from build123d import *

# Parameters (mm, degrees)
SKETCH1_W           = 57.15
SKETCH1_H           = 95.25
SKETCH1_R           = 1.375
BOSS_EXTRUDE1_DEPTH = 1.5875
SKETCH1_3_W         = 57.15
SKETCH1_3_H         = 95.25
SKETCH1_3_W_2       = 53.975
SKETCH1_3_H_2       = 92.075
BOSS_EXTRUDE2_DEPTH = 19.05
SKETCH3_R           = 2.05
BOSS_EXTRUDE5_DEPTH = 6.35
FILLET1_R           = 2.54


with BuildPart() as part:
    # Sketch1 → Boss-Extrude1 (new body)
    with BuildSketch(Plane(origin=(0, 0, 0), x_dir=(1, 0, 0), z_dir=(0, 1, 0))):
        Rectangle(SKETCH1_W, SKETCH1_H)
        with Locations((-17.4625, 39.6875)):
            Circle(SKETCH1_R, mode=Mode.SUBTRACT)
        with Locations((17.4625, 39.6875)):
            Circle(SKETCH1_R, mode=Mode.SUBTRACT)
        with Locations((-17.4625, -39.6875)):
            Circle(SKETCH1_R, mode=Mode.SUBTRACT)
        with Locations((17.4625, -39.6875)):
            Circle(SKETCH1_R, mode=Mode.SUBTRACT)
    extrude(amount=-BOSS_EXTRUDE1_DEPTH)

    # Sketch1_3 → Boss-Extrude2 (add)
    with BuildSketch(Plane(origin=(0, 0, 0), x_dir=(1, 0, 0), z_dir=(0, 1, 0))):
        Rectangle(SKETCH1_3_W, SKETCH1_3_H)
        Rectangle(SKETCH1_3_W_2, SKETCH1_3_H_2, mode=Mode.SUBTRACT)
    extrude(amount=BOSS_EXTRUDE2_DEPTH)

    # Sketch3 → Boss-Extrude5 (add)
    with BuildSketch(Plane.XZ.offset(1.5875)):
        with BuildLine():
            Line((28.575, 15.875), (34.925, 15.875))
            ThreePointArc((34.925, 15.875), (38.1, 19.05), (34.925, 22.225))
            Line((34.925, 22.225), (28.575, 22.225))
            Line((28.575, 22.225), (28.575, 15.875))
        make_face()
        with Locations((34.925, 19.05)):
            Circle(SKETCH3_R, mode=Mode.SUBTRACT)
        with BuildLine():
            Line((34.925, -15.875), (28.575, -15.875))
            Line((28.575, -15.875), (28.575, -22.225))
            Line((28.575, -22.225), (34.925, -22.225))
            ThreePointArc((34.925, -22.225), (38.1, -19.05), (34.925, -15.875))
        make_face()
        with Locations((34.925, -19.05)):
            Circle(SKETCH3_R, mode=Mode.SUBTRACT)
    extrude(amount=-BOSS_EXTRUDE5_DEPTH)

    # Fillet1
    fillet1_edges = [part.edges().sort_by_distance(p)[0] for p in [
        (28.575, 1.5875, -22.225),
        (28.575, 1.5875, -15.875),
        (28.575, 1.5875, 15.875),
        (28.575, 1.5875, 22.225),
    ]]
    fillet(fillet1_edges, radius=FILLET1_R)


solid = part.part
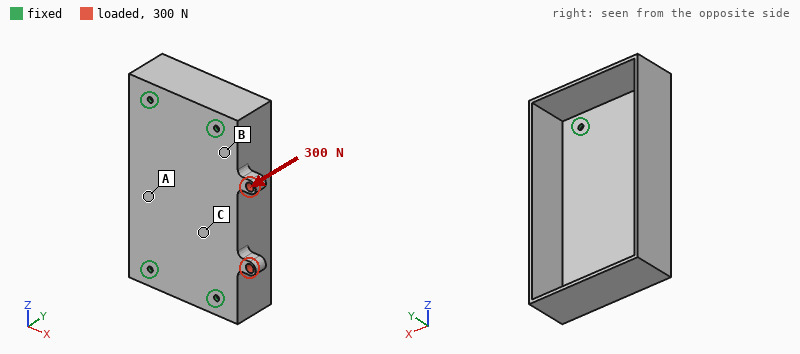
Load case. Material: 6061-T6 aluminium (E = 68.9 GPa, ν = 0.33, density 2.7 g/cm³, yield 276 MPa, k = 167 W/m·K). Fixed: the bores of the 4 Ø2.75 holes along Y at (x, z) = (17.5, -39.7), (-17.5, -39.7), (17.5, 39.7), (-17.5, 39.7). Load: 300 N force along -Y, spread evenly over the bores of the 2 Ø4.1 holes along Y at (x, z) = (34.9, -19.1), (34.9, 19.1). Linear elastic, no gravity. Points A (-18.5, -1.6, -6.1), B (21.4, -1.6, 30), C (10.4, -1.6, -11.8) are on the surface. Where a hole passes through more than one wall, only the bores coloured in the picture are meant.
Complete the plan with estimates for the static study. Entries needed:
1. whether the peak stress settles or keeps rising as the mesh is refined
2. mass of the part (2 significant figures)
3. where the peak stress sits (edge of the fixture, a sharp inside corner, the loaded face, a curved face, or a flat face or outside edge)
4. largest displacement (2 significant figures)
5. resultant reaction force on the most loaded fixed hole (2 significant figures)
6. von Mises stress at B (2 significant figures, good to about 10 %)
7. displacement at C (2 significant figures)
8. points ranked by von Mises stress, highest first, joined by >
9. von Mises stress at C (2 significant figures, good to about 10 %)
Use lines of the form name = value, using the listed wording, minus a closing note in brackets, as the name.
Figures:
whether the peak stress settles or keeps rising as the mesh is refined = keeps rising
mass of the part = 49 g
where the peak stress sits = edge of the fixture
largest displacement = 0.23 mm
resultant reaction force on the most loaded fixed hole = 250 N
von Mises stress at B = 30 MPa
displacement at C = 0.038 mm
points ranked by von Mises stress, highest first, joined by > = B > C > A
von Mises stress at C = 17 MPa
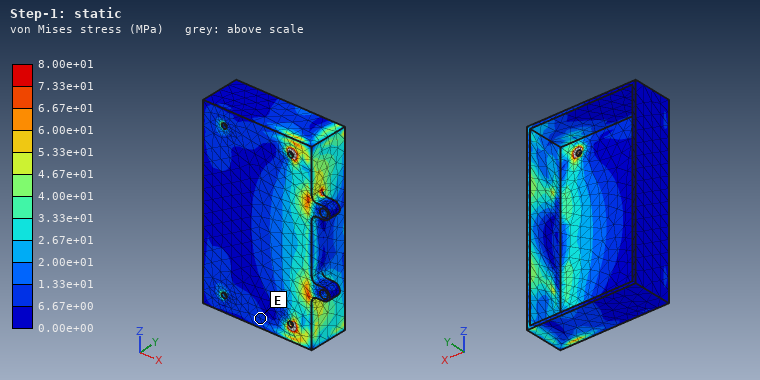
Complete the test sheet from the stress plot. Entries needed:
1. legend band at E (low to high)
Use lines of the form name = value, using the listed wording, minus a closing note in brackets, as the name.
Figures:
legend band at E = 6.67e+00 to 1.33e+01 MPa
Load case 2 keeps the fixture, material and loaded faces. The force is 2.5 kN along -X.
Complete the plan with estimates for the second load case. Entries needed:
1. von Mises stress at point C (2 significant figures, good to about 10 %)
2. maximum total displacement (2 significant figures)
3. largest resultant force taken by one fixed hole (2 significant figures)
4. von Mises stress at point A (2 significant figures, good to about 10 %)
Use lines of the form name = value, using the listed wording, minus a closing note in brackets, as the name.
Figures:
von Mises stress at point C = 29 MPa
maximum total displacement = 0.53 mm
largest resultant force taken by one fixed hole = 700 N
von Mises stress at point A = 16 MPa
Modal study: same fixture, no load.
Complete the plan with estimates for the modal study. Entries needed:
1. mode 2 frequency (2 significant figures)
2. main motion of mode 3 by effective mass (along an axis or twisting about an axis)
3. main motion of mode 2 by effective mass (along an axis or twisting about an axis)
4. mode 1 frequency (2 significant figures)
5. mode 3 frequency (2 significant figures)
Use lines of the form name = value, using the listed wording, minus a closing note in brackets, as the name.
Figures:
mode 2 frequency = 2500 Hz
main motion of mode 3 by effective mass = along Y
main motion of mode 2 by effective mass = along X
mode 1 frequency = 2000 Hz
mode 3 frequency = 3300 Hz
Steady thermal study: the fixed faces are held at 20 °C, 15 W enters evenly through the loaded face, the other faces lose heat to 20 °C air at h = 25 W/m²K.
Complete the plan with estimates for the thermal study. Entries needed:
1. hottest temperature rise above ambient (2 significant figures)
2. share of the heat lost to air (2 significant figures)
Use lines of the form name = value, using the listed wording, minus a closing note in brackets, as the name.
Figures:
hottest temperature rise above ambient = 29 K
share of the heat lost to air = 23 %
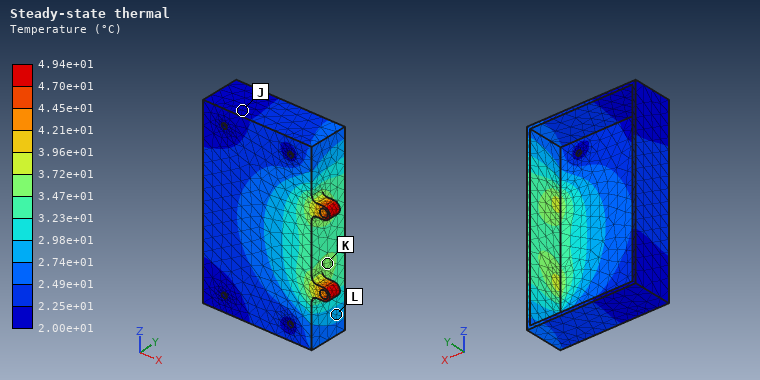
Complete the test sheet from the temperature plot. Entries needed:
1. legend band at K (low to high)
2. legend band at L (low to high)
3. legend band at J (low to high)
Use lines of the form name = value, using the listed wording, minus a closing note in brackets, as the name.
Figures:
legend band at K = 3.47e+01 to 3.72e+01 °C
legend band at L = 2.74e+01 to 2.98e+01 °C
legend band at J = 2.00e+01 to 2.25e+01 °C
